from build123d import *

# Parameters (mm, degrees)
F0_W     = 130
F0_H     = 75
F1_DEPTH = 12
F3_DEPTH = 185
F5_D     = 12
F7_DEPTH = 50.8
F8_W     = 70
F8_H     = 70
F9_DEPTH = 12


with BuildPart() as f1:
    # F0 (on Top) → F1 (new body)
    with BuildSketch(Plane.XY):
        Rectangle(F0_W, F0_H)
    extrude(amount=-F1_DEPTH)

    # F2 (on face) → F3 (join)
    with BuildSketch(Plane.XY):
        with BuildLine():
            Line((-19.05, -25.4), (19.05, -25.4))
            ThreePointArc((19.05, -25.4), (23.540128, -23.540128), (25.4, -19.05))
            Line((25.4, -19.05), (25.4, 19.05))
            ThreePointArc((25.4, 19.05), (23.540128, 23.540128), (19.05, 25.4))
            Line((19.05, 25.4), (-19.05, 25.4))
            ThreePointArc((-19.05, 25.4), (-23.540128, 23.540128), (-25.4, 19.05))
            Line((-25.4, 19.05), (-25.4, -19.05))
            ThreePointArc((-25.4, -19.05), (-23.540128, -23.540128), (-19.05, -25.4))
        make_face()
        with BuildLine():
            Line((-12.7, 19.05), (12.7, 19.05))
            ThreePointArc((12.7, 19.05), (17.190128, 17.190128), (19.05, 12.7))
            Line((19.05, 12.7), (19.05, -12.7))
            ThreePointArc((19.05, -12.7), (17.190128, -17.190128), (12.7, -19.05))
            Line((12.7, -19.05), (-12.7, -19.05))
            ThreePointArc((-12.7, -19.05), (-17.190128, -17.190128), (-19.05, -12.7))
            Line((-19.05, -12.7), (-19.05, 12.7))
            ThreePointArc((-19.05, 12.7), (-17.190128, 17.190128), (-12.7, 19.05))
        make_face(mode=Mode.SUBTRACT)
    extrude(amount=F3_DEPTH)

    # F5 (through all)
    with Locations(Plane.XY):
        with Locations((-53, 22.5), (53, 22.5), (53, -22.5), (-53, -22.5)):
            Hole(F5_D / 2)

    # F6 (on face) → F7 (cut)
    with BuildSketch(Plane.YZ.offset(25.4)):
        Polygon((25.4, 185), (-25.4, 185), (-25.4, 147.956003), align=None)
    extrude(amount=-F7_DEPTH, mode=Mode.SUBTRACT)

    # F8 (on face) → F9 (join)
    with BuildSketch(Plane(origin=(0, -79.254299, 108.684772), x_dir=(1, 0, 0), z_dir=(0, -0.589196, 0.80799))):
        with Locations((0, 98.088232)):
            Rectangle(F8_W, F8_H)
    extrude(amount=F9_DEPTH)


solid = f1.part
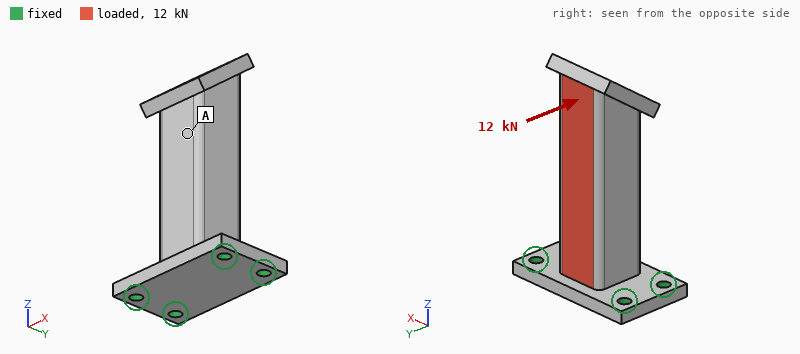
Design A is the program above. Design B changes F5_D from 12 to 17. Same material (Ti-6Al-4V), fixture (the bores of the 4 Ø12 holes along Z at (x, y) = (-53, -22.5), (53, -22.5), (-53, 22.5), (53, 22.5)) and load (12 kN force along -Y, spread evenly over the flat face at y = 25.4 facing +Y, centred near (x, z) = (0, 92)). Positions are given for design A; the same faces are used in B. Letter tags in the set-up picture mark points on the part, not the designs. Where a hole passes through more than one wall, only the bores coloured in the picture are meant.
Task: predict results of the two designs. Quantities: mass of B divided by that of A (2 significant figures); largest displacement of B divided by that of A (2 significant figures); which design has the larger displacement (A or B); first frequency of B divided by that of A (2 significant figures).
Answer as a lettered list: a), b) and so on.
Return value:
a) 0.98
b) 0.87
c) A
d) 1.1
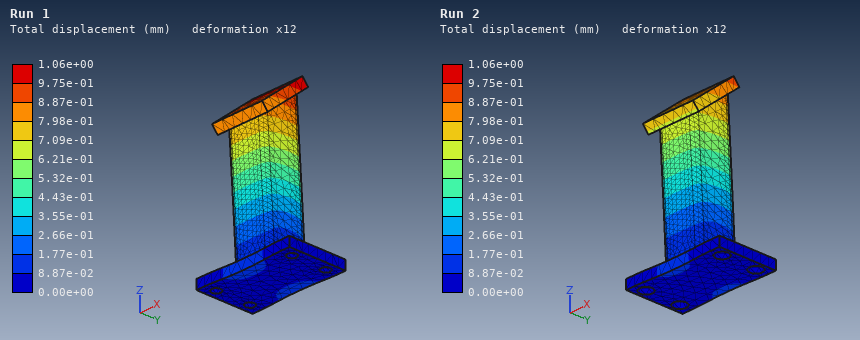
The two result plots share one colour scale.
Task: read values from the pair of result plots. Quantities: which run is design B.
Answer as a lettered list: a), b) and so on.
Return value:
a) Run 2
